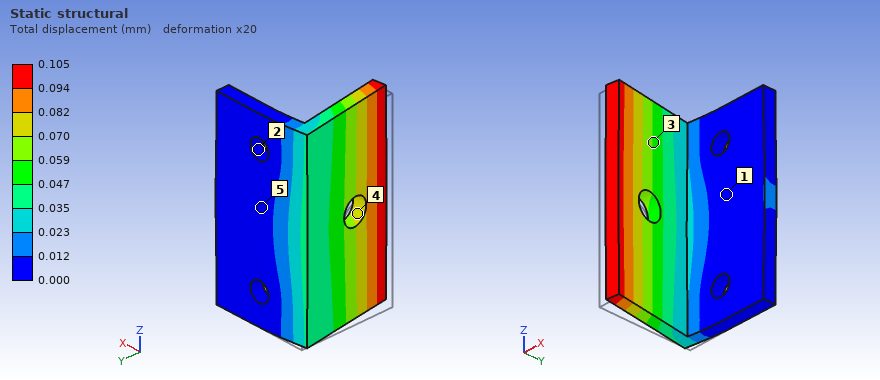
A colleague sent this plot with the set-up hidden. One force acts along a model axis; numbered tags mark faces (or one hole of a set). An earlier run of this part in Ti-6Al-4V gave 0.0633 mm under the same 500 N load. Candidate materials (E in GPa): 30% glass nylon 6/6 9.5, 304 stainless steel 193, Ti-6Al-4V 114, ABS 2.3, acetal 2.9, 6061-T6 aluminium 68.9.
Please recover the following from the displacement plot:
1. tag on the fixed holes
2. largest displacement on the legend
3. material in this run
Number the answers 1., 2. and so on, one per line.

1. 2
2. 0.105 mm
3. 6061-T6 aluminium
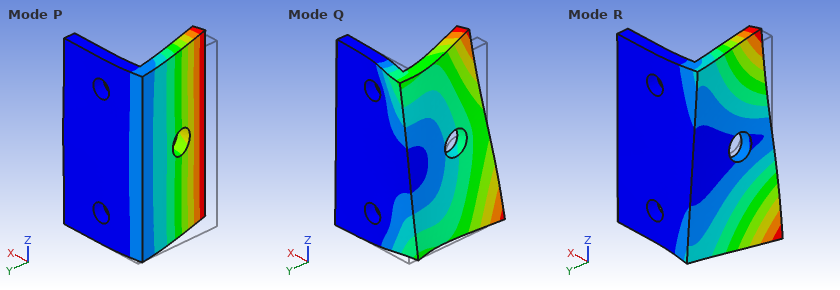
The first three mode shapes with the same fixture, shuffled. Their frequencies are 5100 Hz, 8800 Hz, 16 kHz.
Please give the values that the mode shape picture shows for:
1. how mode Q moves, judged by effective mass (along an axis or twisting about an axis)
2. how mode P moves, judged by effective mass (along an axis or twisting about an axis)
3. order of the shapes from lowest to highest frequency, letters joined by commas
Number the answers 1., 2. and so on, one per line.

1. along Z
2. along X
3. P, R, Q
